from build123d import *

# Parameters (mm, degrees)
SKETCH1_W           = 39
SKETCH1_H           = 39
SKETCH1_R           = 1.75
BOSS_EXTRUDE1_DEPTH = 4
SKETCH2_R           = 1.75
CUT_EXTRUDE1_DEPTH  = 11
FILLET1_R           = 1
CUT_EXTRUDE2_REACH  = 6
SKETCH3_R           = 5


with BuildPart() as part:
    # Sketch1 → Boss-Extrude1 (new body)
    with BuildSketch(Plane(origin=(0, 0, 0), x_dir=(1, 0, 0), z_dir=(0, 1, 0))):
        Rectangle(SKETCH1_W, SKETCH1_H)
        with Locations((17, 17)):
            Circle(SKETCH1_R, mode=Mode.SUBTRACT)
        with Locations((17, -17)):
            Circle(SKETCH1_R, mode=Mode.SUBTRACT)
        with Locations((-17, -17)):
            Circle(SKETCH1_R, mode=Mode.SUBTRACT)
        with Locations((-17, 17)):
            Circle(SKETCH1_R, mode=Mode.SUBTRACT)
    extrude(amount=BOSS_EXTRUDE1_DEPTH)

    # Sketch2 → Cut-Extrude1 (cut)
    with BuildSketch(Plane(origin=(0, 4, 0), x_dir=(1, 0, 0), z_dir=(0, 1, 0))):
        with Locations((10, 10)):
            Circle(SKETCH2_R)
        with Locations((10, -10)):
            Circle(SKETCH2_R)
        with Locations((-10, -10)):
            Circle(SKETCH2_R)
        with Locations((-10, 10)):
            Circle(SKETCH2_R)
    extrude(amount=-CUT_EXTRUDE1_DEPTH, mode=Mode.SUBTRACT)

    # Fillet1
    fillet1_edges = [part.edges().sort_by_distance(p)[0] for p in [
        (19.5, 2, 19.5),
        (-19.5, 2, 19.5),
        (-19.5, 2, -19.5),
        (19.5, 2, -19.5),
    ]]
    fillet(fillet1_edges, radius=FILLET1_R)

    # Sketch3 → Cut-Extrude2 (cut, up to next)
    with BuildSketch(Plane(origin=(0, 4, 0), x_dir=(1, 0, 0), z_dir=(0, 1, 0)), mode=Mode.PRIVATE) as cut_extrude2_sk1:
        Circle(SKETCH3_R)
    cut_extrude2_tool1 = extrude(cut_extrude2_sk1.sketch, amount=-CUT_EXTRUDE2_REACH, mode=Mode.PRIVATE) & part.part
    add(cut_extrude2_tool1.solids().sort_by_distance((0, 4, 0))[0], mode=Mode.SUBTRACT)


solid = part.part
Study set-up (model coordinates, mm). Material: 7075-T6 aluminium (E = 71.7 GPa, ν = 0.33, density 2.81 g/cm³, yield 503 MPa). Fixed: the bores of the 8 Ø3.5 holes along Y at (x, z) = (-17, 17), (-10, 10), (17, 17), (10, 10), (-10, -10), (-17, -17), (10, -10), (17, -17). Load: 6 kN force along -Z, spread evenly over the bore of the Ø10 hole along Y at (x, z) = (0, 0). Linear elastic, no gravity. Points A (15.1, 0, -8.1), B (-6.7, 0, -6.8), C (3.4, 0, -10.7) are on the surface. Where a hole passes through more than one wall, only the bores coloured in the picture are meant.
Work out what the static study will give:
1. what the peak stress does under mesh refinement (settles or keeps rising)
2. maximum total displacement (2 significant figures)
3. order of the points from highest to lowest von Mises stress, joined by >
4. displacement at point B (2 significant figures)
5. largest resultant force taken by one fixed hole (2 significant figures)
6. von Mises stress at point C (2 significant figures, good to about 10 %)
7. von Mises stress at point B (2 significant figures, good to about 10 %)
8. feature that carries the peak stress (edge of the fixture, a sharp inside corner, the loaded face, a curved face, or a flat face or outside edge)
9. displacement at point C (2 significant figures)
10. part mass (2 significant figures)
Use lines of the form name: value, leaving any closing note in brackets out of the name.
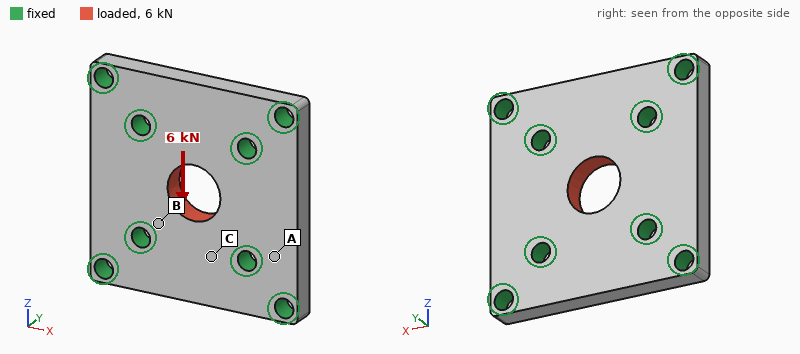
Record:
what the peak stress does under mesh refinement: keeps rising
maximum total displacement: 8.2 µm
order of the points from highest to lowest von Mises stress, joined by >: B > C > A
displacement at point B: 2.8 µm
largest resultant force taken by one fixed hole: 1.5 kN
von Mises stress at point C: 27 MPa
von Mises stress at point B: 48 MPa
feature that carries the peak stress: edge of the fixture
displacement at point C: 4.5 µm
part mass: 15 g
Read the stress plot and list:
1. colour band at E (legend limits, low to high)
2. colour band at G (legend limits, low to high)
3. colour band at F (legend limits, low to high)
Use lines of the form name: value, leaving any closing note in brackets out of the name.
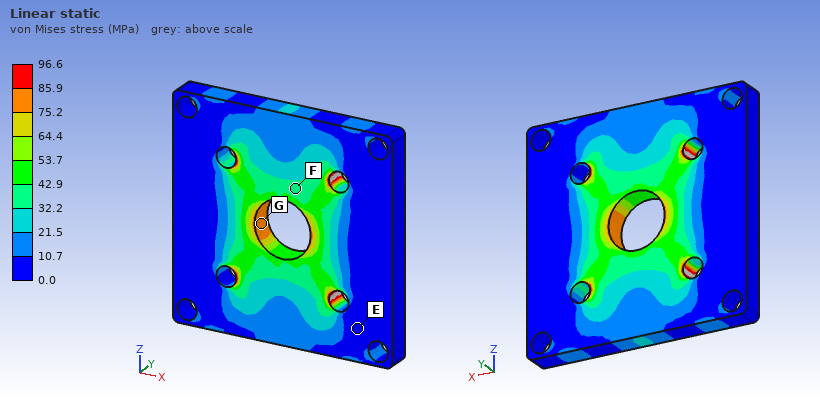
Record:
colour band at E: 0.0 to 10.7 MPa
colour band at G: 75.2 to 85.9 MPa
colour band at F: 32.2 to 42.9 MPa
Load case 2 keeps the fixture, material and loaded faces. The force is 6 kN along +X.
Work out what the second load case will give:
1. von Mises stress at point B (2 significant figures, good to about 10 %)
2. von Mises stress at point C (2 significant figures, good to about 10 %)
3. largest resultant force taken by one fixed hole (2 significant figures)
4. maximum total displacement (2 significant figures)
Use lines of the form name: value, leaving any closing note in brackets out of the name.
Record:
von Mises stress at point B: 48 MPa
von Mises stress at point C: 17 MPa
largest resultant force taken by one fixed hole: 1.5 kN
maximum total displacement: 8.2 µm
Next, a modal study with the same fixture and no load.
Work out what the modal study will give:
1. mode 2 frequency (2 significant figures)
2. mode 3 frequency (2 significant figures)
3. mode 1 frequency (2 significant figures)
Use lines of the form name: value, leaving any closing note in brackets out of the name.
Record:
mode 2 frequency: 34 kHz
mode 3 frequency: 34 kHz
mode 1 frequency: 32 kHz
